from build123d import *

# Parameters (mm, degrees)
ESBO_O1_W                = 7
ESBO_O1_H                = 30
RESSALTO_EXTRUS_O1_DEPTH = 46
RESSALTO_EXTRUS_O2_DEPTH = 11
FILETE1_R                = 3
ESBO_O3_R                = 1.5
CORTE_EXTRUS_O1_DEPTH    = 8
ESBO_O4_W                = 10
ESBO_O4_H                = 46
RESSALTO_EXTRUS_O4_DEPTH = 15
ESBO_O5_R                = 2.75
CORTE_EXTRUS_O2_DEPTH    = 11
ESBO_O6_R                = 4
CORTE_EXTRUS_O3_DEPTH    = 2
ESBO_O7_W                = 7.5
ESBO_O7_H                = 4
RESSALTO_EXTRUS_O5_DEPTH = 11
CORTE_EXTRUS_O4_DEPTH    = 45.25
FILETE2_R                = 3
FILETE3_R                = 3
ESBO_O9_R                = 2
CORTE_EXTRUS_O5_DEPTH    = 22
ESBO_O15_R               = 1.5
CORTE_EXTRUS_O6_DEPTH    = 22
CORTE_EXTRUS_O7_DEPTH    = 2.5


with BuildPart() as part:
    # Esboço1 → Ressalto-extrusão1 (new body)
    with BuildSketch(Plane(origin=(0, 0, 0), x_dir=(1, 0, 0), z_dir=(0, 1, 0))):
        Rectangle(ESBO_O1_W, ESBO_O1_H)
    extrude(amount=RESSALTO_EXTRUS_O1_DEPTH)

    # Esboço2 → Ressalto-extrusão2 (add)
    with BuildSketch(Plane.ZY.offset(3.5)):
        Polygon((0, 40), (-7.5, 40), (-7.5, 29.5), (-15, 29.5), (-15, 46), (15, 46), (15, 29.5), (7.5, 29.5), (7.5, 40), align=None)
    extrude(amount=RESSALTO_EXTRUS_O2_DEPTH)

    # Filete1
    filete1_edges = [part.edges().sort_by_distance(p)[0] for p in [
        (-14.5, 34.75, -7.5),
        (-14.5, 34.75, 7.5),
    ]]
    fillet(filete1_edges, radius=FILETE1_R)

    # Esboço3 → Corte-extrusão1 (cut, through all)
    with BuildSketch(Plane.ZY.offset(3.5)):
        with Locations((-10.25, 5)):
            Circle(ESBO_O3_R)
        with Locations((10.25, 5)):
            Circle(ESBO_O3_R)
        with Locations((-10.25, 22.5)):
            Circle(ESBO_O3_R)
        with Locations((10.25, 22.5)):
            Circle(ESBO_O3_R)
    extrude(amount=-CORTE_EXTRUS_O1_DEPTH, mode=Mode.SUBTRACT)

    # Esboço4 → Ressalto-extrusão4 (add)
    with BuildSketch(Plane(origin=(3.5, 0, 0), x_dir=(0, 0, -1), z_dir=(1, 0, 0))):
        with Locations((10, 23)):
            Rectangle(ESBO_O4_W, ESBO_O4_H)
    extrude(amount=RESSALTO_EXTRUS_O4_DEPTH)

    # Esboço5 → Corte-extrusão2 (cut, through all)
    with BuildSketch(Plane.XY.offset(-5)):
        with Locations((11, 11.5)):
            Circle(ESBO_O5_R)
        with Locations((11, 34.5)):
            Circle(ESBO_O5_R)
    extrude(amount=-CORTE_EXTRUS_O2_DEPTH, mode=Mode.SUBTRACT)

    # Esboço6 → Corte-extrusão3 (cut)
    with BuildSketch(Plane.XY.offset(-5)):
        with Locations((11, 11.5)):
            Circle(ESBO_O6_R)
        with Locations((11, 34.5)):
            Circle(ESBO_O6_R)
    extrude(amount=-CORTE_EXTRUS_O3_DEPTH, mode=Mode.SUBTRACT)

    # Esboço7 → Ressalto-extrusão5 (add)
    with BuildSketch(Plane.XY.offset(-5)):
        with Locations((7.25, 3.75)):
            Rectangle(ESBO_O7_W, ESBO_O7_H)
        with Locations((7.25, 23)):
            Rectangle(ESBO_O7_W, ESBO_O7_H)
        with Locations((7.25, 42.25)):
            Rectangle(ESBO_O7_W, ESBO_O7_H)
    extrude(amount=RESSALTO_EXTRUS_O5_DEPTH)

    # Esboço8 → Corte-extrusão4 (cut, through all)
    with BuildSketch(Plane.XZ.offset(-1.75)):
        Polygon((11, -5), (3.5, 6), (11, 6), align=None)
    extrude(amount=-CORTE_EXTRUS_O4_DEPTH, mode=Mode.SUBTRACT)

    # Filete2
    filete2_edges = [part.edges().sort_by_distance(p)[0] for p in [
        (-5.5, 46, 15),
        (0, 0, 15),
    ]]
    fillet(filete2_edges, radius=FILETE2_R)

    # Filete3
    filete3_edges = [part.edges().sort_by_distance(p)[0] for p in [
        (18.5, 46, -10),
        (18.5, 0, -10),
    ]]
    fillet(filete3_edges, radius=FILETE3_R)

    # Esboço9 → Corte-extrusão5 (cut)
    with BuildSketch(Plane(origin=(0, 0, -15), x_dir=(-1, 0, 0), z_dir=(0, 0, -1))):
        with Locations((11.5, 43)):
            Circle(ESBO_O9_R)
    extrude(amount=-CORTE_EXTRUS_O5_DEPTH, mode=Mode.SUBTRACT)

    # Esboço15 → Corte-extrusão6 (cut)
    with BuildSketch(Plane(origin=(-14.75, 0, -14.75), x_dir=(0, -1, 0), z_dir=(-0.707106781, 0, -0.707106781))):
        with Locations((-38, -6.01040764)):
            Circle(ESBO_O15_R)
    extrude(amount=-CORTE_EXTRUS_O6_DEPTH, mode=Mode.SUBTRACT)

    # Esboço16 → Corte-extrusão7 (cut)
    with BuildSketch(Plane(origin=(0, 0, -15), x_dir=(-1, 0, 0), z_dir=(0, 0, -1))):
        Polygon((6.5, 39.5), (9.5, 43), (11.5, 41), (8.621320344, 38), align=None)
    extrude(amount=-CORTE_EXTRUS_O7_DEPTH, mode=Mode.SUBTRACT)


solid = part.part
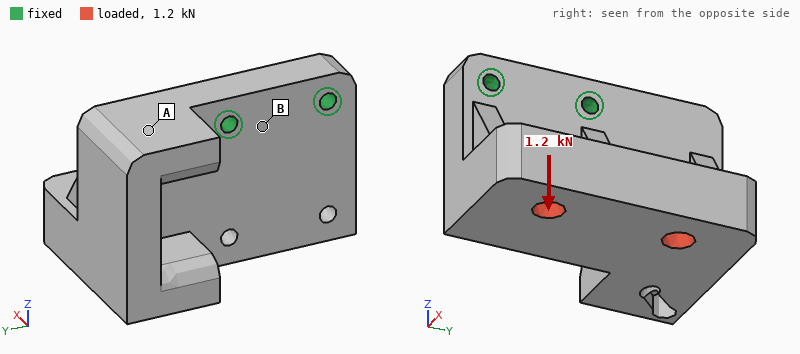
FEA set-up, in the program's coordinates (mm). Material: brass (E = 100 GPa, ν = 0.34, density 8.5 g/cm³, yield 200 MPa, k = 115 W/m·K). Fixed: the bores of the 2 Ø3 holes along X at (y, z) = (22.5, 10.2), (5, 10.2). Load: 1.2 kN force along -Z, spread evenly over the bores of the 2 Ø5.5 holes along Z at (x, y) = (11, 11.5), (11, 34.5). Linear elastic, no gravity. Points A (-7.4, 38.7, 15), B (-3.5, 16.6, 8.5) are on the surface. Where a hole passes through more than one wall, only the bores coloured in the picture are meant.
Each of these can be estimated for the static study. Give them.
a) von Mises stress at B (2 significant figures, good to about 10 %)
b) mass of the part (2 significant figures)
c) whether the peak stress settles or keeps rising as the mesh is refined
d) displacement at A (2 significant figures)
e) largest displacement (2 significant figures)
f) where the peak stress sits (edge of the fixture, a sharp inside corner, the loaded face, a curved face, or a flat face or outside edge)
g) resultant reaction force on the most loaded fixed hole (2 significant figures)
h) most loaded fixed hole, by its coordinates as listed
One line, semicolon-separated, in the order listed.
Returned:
21 MPa; 170 g; keeps rising; 11 µm; 51 µm; edge of the fixture; 1.2 kN; (22.5, 10.2)
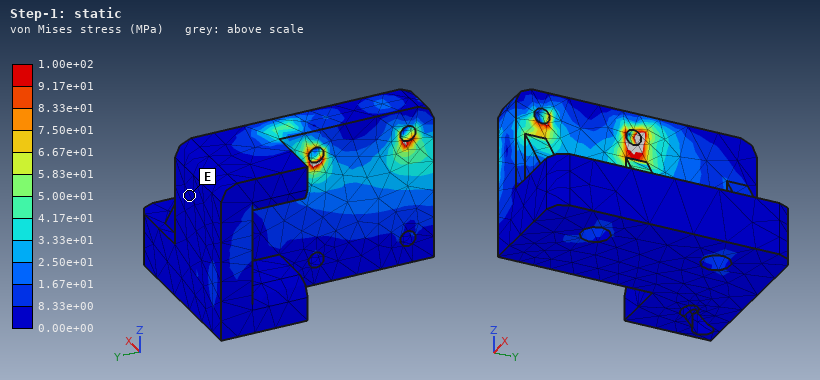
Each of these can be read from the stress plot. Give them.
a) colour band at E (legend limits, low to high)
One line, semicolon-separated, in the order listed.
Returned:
0.00e+00 to 8.33e+00 MPa
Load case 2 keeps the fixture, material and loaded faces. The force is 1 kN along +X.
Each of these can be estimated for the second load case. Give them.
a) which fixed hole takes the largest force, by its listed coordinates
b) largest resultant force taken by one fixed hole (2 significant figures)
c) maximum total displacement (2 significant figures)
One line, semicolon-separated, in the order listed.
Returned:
(22.5, 10.2); 870 N; 72 µm
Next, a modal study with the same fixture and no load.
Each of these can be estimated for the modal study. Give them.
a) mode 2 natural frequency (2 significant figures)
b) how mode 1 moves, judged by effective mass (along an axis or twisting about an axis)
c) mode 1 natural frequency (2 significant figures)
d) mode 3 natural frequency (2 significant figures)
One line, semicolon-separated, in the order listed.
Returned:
3600 Hz; along X; 2100 Hz; 4800 Hz
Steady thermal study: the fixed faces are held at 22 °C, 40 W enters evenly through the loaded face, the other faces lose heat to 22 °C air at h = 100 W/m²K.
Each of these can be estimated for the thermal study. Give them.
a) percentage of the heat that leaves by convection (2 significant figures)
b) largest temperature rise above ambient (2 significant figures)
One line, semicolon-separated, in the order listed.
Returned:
28 %; 28 K
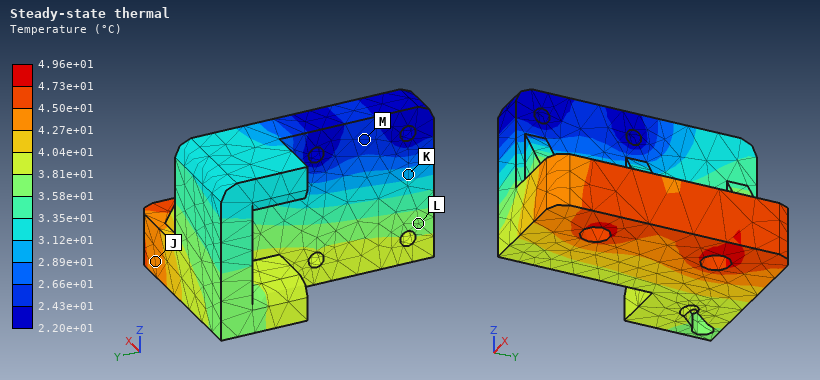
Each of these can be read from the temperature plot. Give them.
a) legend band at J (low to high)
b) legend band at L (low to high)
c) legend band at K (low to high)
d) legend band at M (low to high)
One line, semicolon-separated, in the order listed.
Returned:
4.27e+01 to 4.50e+01 °C; 3.58e+01 to 3.81e+01 °C; 2.89e+01 to 3.12e+01 °C; 2.43e+01 to 2.66e+01 °C
